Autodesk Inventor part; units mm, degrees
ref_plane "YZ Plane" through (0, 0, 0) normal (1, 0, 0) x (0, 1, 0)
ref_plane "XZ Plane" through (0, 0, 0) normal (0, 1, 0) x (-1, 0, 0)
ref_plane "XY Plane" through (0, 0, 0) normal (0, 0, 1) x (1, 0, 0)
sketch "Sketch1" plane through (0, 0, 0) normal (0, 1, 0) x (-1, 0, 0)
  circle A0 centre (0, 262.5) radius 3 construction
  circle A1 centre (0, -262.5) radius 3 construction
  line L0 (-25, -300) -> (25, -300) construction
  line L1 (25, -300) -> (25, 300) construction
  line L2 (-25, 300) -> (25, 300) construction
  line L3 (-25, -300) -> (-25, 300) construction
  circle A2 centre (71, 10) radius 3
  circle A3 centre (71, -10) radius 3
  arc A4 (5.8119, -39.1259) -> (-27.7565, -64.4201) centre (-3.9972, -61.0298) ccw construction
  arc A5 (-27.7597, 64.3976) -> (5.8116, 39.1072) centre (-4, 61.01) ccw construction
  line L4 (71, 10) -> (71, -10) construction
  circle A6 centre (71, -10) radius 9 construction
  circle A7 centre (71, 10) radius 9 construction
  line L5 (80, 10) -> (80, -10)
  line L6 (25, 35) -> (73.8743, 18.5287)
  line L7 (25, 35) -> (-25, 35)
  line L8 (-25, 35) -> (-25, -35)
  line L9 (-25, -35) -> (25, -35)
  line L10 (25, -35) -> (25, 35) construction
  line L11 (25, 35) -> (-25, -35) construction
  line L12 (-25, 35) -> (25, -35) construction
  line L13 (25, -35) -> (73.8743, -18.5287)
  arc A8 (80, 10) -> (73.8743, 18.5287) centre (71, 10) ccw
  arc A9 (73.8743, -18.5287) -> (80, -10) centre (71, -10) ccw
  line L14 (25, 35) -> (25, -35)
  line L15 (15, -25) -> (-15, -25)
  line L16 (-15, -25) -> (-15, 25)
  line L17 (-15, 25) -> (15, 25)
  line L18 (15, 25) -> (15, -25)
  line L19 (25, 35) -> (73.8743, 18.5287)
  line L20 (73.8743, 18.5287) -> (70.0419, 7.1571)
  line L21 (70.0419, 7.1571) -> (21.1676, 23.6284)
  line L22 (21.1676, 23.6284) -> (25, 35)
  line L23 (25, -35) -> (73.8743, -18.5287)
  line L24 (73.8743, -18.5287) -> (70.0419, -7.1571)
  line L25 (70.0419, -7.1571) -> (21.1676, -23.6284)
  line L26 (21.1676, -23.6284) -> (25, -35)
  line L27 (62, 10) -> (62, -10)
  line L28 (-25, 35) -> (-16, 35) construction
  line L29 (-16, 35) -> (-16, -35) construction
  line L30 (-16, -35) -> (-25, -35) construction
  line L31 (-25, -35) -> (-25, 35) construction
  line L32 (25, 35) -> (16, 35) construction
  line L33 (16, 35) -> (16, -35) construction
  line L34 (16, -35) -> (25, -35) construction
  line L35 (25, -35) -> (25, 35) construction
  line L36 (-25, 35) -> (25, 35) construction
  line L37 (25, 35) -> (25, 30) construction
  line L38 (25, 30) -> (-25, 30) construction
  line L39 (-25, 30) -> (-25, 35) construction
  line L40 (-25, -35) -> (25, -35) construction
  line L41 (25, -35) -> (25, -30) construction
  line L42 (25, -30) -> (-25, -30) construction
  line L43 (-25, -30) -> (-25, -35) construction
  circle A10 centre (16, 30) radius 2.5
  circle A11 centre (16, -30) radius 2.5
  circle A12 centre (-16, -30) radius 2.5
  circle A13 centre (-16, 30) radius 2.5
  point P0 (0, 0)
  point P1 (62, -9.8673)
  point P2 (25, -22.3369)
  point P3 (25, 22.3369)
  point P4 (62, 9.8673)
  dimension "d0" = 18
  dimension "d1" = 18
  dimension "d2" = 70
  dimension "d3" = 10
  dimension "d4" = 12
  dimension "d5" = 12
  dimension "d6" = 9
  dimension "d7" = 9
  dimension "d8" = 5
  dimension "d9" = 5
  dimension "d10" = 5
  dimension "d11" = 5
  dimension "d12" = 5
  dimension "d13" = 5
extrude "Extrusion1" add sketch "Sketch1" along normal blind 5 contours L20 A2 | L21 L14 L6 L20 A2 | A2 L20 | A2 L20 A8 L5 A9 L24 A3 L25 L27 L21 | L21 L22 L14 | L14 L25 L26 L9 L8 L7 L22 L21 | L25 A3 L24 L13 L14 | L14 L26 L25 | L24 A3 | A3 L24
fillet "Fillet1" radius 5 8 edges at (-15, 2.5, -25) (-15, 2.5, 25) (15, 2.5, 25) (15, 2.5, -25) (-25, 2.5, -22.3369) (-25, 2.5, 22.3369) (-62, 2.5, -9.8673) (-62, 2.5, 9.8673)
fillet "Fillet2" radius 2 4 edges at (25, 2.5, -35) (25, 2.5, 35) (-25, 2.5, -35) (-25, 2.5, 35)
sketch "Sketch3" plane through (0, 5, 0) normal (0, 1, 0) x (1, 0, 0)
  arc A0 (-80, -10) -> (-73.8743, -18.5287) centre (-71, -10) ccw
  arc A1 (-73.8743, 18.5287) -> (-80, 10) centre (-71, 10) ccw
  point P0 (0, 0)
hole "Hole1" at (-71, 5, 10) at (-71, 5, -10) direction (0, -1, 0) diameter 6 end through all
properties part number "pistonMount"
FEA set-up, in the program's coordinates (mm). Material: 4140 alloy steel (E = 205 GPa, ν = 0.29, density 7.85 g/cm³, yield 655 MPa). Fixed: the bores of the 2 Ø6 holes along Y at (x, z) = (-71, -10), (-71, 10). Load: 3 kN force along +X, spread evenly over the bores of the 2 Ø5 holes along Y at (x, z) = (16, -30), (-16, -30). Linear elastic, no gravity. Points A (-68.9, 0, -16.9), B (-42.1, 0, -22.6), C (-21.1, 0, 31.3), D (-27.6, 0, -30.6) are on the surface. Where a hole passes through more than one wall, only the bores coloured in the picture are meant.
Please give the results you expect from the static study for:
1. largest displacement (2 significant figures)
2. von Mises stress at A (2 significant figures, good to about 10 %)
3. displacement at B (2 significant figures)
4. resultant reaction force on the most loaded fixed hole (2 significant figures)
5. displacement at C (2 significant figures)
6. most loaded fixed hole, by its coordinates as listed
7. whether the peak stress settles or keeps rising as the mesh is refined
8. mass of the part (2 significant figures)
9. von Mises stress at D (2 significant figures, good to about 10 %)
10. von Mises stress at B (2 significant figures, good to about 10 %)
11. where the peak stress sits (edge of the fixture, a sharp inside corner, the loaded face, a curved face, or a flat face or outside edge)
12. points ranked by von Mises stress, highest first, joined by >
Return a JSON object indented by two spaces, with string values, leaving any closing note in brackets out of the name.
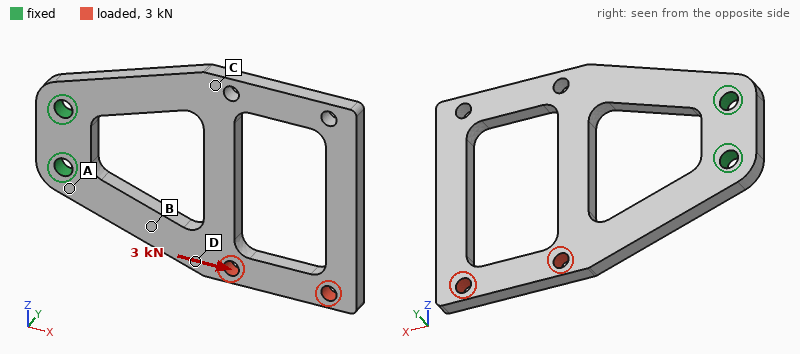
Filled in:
{
  "largest displacement": "0.17 mm",
  "von Mises stress at A": "110 MPa",
  "displacement at B": "0.050 mm",
  "resultant reaction force on the most loaded fixed hole": "4.6 kN",
  "displacement at C": "0.089 mm",
  "most loaded fixed hole, by its coordinates as listed": "(-71, -10)",
  "whether the peak stress settles or keeps rising as the mesh is refined": "keeps rising",
  "mass of the part": "140 g",
  "von Mises stress at D": "37 MPa",
  "von Mises stress at B": "63 MPa",
  "where the peak stress sits": "edge of the fixture",
  "points ranked by von Mises stress, highest first, joined by >": "A > B > D > C"
}
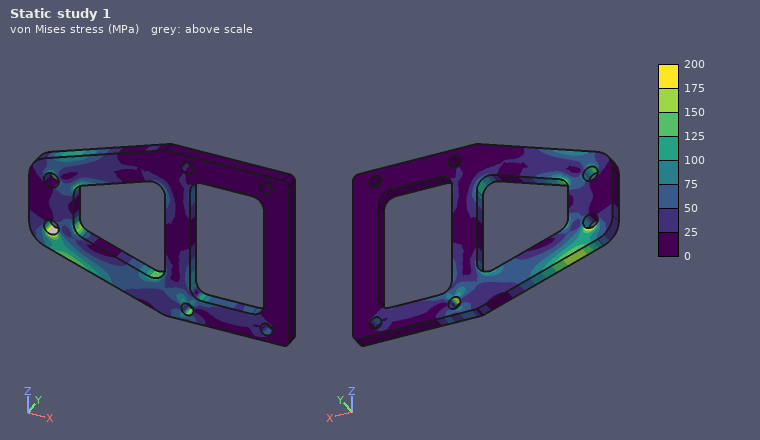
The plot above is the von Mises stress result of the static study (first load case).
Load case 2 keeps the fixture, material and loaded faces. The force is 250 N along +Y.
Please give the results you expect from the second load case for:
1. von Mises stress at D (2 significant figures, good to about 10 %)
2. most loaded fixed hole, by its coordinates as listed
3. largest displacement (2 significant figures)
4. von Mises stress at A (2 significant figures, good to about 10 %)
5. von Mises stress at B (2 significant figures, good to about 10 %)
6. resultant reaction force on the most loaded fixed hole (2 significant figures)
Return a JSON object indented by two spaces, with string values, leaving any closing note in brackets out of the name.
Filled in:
{
  "von Mises stress at D": "54 MPa",
  "most loaded fixed hole, by its coordinates as listed": "(-71, -10)",
  "largest displacement": "1.1 mm",
  "von Mises stress at A": "150 MPa",
  "von Mises stress at B": "120 MPa",
  "resultant reaction force on the most loaded fixed hole": "280 N"
}
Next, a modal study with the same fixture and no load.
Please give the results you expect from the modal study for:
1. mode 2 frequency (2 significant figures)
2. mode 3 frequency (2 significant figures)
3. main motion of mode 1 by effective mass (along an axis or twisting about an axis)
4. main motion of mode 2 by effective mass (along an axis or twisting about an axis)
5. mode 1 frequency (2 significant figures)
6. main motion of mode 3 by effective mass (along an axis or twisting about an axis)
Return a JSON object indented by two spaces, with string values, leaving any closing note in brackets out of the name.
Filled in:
{
  "mode 2 frequency": "910 Hz",
  "mode 3 frequency": "1300 Hz",
  "main motion of mode 1 by effective mass": "along Y",
  "main motion of mode 2 by effective mass": "twisting about X",
  "mode 1 frequency": "350 Hz",
  "main motion of mode 3 by effective mass": "along Z"
}
